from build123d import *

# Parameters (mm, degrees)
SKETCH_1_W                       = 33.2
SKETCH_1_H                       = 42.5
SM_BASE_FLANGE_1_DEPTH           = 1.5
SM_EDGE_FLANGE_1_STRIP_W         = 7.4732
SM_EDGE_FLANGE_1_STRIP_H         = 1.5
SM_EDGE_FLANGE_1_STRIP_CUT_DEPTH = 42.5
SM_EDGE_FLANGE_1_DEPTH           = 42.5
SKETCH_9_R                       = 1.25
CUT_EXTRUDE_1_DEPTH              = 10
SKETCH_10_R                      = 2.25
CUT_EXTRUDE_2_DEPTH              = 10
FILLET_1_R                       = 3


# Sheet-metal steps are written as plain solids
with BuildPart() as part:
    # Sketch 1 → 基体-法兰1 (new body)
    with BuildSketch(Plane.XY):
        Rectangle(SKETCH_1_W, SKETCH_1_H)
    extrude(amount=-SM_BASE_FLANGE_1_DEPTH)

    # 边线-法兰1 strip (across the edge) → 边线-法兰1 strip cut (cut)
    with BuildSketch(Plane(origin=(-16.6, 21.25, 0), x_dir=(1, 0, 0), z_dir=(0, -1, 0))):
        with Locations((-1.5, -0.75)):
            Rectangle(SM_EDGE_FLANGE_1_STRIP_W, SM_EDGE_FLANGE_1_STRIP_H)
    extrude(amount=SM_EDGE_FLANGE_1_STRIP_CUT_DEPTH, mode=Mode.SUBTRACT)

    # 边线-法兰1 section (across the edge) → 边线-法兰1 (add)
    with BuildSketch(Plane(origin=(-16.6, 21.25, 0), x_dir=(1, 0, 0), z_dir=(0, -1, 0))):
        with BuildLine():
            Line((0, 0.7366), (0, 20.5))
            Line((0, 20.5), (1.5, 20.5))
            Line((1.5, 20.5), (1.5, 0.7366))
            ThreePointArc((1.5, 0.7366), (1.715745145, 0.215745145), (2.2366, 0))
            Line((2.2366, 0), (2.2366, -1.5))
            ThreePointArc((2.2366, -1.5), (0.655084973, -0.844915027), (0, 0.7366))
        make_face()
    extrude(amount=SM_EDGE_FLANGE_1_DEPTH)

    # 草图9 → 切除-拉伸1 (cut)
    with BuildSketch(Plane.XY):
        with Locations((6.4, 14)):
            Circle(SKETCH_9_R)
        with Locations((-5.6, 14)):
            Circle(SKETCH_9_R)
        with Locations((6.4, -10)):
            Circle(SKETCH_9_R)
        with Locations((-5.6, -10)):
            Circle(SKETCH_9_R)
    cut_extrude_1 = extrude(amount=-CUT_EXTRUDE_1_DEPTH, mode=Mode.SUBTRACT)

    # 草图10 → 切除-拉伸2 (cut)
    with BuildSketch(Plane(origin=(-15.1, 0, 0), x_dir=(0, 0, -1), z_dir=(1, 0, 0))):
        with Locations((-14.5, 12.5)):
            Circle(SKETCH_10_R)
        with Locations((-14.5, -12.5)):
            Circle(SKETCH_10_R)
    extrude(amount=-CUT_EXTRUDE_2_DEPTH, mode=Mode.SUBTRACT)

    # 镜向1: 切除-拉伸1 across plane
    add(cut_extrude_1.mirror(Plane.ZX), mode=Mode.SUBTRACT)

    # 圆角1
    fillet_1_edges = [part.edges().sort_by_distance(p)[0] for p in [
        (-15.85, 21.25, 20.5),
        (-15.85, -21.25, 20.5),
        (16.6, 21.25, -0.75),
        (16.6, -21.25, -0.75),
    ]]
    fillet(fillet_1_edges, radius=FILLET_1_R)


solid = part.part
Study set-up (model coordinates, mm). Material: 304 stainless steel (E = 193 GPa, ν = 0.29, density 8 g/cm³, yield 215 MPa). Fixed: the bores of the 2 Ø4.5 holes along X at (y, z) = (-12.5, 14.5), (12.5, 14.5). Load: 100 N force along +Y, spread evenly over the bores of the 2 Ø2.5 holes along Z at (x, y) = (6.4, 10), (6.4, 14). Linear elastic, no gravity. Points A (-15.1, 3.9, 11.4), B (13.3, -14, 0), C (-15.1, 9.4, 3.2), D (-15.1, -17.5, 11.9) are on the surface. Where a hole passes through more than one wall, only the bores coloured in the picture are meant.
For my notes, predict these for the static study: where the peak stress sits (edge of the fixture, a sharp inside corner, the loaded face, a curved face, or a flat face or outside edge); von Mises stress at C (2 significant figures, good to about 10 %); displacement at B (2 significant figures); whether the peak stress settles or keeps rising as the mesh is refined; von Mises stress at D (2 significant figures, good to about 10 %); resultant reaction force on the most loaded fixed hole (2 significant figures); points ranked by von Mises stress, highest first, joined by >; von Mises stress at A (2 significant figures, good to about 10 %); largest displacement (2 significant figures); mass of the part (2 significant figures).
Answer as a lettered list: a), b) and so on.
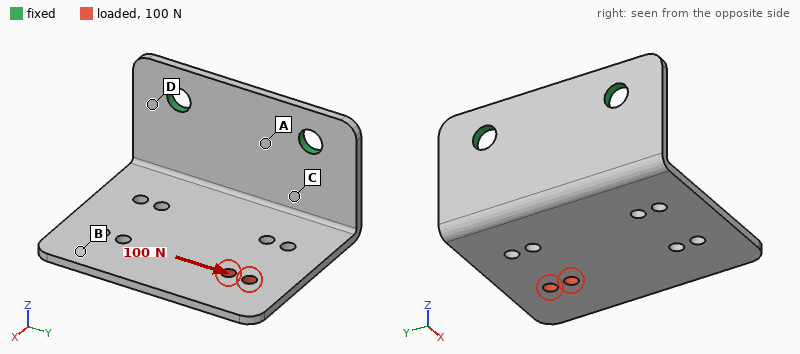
a) edge of the fixture
b) 49 MPa
c) 0.089 mm
d) keeps rising
e) 68 MPa
f) 110 N
g) D > C > A > B
h) 24 MPa
i) 0.11 mm
j) 26 g
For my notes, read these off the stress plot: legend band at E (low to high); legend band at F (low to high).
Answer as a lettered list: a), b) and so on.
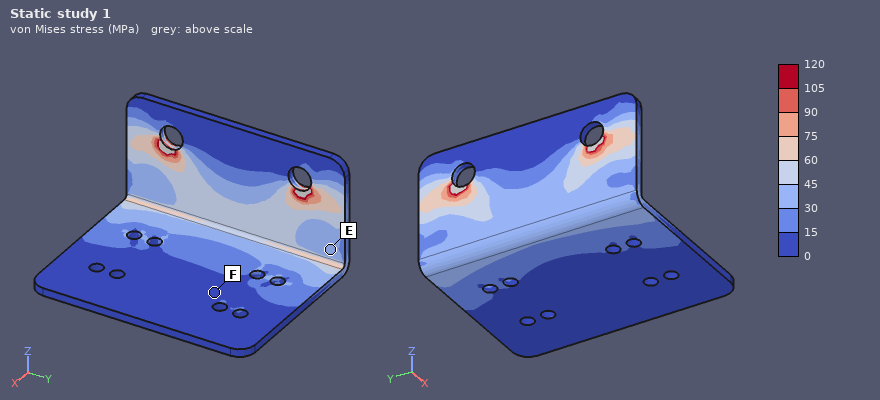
a) 30 to 45 MPa
b) 0 to 15 MPa
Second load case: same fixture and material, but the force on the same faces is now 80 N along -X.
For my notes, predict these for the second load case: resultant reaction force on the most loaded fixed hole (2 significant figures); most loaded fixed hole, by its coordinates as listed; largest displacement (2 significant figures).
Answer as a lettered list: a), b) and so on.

a) 73 N
b) (12.5, 14.5)
c) 0.15 mm
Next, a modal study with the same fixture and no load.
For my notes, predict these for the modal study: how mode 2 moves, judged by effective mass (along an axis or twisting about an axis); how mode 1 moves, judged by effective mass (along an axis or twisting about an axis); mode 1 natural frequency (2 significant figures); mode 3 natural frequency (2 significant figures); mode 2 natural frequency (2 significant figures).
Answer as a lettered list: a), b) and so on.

a) along Y
b) along Z
c) 680 Hz
d) 2300 Hz
e) 1500 Hz
